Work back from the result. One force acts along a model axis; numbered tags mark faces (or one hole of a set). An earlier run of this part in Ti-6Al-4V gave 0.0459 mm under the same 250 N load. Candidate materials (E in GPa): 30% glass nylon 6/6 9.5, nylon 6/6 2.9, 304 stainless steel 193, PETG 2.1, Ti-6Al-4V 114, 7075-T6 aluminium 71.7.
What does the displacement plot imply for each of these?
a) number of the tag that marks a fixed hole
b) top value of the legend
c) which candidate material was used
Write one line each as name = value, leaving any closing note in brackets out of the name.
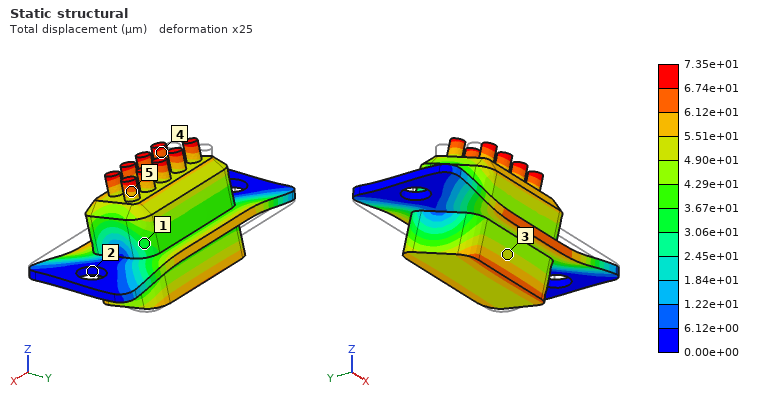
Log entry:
number of the tag that marks a fixed hole = 2
top value of the legend = 7.35e+01 µm
which candidate material was used = 7075-T6 aluminium
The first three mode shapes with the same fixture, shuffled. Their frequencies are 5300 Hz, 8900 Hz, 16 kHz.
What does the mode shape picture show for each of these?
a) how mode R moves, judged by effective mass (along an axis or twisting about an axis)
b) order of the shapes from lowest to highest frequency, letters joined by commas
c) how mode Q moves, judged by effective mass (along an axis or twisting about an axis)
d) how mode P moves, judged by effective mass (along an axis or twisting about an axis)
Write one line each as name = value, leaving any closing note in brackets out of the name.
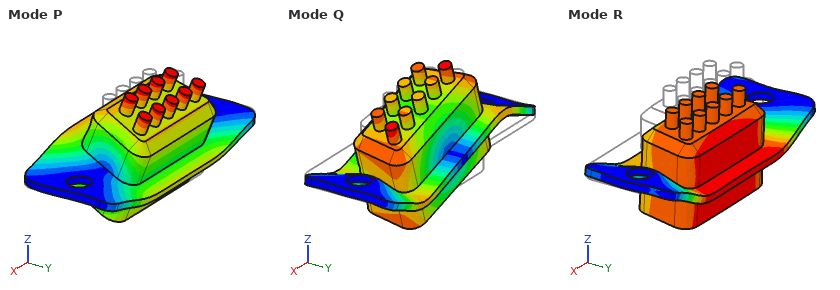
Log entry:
how mode R moves, judged by effective mass = along Z
order of the shapes from lowest to highest frequency, letters joined by commas = P, R, Q
how mode Q moves, judged by effective mass = twisting about Y
how mode P moves, judged by effective mass = twisting about X
